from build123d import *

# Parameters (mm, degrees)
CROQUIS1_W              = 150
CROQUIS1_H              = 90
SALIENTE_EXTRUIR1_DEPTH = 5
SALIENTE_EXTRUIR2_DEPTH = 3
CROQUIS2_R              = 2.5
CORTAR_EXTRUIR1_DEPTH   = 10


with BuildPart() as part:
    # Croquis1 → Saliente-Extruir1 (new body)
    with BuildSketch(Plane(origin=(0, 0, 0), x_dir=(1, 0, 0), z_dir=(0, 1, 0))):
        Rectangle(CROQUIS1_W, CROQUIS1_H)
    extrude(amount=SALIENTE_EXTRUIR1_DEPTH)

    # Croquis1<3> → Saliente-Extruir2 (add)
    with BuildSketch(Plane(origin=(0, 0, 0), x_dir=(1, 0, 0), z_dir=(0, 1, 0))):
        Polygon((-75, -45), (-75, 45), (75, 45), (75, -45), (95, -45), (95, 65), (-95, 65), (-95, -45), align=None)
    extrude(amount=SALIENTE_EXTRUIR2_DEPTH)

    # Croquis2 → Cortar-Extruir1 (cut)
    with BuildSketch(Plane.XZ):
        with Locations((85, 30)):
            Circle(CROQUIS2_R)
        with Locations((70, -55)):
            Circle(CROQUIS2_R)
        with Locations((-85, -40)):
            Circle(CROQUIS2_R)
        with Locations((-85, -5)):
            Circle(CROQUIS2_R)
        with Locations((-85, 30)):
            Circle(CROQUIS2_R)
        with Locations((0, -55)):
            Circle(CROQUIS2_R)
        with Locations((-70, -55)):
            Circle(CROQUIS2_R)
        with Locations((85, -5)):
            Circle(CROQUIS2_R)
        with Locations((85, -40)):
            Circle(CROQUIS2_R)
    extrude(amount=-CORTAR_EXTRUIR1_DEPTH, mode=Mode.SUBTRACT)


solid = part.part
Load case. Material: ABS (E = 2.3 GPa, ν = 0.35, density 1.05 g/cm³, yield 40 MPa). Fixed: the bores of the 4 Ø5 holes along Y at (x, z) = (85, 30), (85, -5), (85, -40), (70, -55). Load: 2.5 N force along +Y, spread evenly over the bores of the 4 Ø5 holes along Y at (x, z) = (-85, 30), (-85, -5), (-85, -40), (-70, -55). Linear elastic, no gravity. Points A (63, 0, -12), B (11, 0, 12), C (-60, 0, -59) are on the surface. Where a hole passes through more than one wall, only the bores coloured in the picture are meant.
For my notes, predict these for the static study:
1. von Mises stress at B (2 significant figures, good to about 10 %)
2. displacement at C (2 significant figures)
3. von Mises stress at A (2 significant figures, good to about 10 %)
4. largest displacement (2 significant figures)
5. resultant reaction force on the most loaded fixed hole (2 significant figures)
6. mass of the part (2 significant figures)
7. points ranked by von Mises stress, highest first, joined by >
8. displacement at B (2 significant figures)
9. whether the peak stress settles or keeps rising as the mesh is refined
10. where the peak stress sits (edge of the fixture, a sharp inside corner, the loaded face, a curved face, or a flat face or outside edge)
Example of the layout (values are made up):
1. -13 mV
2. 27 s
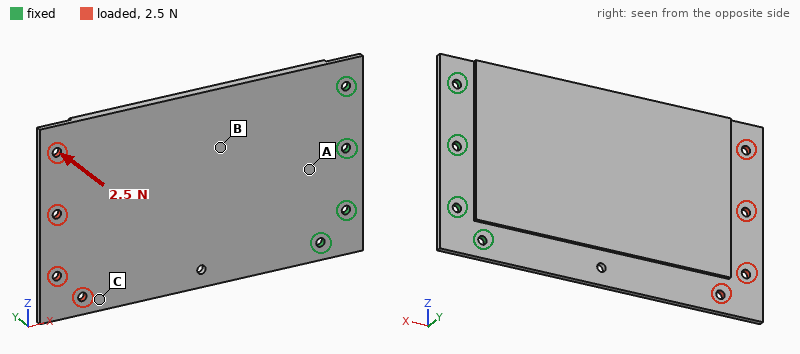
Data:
1. 0.55 MPa
2. 1.7 mm
3. 0.73 MPa
4. 2.4 mm
5. 14 N
6. 94 g
7. A > B > C
8. 0.65 mm
9. keeps rising
10. edge of the fixture
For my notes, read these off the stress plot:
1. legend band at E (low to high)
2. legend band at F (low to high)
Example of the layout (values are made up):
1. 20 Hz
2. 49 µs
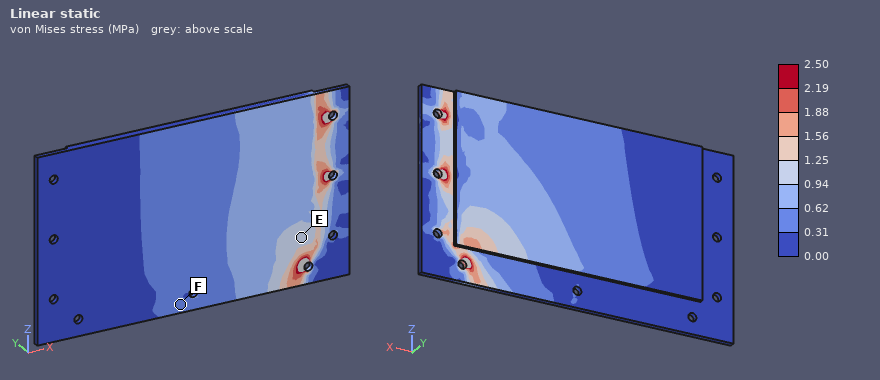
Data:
1. 0.94 to 1.25 MPa
2. 0.31 to 0.62 MPa
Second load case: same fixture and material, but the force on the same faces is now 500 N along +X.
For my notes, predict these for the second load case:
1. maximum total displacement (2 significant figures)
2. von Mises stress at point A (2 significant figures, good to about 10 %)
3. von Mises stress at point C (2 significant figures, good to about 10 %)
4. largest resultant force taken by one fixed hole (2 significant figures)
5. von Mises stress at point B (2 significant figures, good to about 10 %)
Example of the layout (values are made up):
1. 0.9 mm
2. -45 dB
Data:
1. 2.3 mm
2. 1.7 MPa
3. 2.8 MPa
4. 140 N
5. 1.7 MPa
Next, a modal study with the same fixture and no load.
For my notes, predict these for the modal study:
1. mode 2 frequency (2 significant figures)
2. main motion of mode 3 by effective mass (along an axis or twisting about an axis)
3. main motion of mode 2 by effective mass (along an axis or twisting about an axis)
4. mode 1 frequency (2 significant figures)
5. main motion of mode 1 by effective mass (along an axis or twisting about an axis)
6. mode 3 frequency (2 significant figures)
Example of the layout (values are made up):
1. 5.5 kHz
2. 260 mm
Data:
1. 130 Hz
2. along Y
3. twisting about X
4. 33 Hz
5. along Y
6. 220 Hz
